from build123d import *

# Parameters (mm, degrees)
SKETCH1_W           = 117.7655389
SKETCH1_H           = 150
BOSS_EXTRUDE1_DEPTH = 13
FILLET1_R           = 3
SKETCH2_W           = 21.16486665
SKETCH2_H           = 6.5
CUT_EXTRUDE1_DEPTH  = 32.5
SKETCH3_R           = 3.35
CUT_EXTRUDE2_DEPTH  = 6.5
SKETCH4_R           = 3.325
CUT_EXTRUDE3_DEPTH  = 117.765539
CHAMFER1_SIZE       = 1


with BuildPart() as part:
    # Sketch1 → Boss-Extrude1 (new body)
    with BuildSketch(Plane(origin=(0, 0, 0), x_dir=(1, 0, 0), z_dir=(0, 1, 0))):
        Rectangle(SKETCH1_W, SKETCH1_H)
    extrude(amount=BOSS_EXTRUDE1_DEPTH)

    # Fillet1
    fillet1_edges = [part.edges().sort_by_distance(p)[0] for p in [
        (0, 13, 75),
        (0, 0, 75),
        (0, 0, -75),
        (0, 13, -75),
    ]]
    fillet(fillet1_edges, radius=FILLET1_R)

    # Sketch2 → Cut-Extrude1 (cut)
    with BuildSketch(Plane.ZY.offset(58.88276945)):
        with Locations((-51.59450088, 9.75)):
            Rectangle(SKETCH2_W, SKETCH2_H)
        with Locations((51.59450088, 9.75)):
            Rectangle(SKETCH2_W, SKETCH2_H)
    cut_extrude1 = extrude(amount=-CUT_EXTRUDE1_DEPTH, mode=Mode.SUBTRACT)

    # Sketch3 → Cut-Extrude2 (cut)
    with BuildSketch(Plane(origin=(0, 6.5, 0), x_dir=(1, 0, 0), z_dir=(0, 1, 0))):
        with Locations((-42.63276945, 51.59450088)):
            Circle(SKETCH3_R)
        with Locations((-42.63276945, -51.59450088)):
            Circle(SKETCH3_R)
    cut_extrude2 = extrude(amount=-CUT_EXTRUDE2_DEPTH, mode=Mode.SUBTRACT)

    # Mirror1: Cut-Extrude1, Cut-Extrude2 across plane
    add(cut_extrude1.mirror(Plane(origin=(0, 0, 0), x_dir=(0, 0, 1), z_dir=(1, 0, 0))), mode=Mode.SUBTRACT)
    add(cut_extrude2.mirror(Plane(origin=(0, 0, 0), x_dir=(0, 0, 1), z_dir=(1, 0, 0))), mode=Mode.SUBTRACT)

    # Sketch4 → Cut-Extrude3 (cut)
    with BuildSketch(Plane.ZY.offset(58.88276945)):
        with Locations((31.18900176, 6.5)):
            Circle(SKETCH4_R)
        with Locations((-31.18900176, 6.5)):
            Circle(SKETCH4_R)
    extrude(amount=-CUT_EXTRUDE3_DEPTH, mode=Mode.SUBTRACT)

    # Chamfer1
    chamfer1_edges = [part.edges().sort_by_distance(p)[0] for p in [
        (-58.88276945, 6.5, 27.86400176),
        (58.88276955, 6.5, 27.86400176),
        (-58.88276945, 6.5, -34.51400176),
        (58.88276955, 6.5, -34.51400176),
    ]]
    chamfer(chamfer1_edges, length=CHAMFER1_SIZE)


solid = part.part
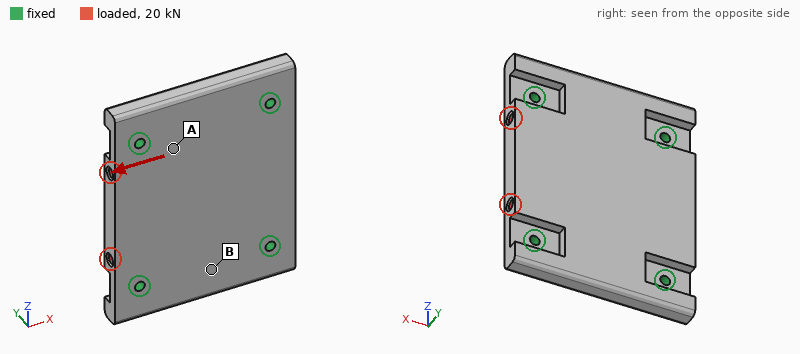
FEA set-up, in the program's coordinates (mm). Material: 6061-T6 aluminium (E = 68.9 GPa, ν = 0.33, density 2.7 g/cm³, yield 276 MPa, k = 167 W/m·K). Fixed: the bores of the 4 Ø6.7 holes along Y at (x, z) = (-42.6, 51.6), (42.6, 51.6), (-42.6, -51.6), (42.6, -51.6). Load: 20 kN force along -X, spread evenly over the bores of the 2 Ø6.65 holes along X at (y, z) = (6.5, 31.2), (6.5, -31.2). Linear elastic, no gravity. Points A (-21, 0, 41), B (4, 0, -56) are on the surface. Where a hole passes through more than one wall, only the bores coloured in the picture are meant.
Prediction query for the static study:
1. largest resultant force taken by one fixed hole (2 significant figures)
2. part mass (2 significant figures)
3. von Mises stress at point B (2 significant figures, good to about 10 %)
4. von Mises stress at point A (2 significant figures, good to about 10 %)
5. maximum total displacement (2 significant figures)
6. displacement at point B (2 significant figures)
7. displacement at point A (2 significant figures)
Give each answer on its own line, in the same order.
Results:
5.2 kN
540 g
6.9 MPa
17 MPa
15 µm
6.8 µm
9.2 µm
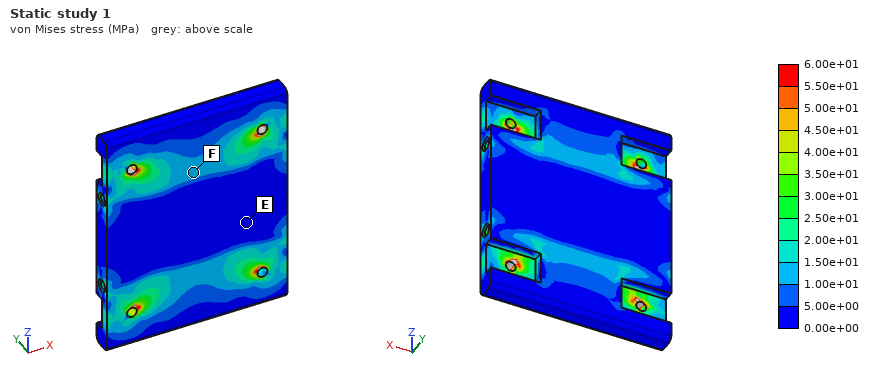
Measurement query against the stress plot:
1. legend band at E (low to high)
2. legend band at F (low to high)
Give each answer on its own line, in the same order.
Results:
0.00e+00 to 5.00e+00 MPa
1.00e+01 to 1.50e+01 MPa
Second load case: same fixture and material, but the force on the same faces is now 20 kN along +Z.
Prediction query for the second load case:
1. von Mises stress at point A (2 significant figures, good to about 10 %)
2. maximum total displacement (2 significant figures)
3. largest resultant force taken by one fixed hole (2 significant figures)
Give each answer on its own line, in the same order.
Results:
8.3 MPa
13 µm
5.0 kN
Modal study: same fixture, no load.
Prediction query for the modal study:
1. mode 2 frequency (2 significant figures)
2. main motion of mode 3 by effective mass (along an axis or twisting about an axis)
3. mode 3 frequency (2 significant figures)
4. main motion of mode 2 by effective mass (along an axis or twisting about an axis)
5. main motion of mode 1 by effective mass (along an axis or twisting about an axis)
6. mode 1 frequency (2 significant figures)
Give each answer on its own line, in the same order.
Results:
4700 Hz
along Y
4900 Hz
twisting about Z
along Y
3400 Hz
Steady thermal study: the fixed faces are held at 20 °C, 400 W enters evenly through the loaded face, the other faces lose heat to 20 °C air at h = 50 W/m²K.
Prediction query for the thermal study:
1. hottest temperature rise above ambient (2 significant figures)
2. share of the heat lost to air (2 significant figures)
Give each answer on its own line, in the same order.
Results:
41 K
15 %
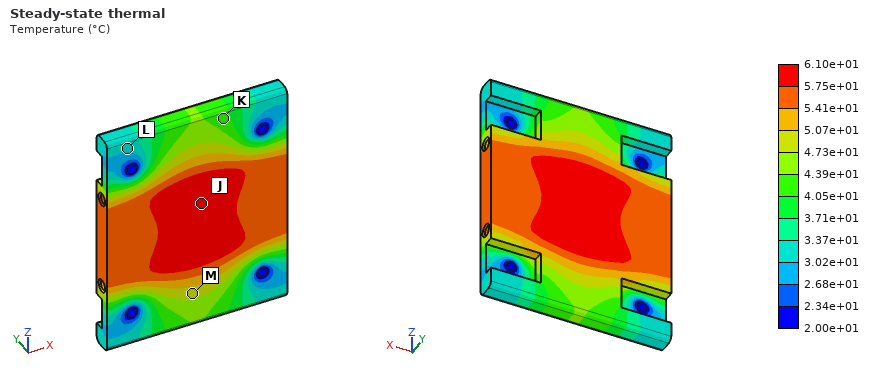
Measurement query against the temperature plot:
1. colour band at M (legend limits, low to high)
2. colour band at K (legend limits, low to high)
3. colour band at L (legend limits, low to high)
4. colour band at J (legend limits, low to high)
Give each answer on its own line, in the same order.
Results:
4.73e+01 to 5.07e+01 °C
4.05e+01 to 4.39e+01 °C
3.02e+01 to 3.37e+01 °C
5.75e+01 to 6.10e+01 °C
